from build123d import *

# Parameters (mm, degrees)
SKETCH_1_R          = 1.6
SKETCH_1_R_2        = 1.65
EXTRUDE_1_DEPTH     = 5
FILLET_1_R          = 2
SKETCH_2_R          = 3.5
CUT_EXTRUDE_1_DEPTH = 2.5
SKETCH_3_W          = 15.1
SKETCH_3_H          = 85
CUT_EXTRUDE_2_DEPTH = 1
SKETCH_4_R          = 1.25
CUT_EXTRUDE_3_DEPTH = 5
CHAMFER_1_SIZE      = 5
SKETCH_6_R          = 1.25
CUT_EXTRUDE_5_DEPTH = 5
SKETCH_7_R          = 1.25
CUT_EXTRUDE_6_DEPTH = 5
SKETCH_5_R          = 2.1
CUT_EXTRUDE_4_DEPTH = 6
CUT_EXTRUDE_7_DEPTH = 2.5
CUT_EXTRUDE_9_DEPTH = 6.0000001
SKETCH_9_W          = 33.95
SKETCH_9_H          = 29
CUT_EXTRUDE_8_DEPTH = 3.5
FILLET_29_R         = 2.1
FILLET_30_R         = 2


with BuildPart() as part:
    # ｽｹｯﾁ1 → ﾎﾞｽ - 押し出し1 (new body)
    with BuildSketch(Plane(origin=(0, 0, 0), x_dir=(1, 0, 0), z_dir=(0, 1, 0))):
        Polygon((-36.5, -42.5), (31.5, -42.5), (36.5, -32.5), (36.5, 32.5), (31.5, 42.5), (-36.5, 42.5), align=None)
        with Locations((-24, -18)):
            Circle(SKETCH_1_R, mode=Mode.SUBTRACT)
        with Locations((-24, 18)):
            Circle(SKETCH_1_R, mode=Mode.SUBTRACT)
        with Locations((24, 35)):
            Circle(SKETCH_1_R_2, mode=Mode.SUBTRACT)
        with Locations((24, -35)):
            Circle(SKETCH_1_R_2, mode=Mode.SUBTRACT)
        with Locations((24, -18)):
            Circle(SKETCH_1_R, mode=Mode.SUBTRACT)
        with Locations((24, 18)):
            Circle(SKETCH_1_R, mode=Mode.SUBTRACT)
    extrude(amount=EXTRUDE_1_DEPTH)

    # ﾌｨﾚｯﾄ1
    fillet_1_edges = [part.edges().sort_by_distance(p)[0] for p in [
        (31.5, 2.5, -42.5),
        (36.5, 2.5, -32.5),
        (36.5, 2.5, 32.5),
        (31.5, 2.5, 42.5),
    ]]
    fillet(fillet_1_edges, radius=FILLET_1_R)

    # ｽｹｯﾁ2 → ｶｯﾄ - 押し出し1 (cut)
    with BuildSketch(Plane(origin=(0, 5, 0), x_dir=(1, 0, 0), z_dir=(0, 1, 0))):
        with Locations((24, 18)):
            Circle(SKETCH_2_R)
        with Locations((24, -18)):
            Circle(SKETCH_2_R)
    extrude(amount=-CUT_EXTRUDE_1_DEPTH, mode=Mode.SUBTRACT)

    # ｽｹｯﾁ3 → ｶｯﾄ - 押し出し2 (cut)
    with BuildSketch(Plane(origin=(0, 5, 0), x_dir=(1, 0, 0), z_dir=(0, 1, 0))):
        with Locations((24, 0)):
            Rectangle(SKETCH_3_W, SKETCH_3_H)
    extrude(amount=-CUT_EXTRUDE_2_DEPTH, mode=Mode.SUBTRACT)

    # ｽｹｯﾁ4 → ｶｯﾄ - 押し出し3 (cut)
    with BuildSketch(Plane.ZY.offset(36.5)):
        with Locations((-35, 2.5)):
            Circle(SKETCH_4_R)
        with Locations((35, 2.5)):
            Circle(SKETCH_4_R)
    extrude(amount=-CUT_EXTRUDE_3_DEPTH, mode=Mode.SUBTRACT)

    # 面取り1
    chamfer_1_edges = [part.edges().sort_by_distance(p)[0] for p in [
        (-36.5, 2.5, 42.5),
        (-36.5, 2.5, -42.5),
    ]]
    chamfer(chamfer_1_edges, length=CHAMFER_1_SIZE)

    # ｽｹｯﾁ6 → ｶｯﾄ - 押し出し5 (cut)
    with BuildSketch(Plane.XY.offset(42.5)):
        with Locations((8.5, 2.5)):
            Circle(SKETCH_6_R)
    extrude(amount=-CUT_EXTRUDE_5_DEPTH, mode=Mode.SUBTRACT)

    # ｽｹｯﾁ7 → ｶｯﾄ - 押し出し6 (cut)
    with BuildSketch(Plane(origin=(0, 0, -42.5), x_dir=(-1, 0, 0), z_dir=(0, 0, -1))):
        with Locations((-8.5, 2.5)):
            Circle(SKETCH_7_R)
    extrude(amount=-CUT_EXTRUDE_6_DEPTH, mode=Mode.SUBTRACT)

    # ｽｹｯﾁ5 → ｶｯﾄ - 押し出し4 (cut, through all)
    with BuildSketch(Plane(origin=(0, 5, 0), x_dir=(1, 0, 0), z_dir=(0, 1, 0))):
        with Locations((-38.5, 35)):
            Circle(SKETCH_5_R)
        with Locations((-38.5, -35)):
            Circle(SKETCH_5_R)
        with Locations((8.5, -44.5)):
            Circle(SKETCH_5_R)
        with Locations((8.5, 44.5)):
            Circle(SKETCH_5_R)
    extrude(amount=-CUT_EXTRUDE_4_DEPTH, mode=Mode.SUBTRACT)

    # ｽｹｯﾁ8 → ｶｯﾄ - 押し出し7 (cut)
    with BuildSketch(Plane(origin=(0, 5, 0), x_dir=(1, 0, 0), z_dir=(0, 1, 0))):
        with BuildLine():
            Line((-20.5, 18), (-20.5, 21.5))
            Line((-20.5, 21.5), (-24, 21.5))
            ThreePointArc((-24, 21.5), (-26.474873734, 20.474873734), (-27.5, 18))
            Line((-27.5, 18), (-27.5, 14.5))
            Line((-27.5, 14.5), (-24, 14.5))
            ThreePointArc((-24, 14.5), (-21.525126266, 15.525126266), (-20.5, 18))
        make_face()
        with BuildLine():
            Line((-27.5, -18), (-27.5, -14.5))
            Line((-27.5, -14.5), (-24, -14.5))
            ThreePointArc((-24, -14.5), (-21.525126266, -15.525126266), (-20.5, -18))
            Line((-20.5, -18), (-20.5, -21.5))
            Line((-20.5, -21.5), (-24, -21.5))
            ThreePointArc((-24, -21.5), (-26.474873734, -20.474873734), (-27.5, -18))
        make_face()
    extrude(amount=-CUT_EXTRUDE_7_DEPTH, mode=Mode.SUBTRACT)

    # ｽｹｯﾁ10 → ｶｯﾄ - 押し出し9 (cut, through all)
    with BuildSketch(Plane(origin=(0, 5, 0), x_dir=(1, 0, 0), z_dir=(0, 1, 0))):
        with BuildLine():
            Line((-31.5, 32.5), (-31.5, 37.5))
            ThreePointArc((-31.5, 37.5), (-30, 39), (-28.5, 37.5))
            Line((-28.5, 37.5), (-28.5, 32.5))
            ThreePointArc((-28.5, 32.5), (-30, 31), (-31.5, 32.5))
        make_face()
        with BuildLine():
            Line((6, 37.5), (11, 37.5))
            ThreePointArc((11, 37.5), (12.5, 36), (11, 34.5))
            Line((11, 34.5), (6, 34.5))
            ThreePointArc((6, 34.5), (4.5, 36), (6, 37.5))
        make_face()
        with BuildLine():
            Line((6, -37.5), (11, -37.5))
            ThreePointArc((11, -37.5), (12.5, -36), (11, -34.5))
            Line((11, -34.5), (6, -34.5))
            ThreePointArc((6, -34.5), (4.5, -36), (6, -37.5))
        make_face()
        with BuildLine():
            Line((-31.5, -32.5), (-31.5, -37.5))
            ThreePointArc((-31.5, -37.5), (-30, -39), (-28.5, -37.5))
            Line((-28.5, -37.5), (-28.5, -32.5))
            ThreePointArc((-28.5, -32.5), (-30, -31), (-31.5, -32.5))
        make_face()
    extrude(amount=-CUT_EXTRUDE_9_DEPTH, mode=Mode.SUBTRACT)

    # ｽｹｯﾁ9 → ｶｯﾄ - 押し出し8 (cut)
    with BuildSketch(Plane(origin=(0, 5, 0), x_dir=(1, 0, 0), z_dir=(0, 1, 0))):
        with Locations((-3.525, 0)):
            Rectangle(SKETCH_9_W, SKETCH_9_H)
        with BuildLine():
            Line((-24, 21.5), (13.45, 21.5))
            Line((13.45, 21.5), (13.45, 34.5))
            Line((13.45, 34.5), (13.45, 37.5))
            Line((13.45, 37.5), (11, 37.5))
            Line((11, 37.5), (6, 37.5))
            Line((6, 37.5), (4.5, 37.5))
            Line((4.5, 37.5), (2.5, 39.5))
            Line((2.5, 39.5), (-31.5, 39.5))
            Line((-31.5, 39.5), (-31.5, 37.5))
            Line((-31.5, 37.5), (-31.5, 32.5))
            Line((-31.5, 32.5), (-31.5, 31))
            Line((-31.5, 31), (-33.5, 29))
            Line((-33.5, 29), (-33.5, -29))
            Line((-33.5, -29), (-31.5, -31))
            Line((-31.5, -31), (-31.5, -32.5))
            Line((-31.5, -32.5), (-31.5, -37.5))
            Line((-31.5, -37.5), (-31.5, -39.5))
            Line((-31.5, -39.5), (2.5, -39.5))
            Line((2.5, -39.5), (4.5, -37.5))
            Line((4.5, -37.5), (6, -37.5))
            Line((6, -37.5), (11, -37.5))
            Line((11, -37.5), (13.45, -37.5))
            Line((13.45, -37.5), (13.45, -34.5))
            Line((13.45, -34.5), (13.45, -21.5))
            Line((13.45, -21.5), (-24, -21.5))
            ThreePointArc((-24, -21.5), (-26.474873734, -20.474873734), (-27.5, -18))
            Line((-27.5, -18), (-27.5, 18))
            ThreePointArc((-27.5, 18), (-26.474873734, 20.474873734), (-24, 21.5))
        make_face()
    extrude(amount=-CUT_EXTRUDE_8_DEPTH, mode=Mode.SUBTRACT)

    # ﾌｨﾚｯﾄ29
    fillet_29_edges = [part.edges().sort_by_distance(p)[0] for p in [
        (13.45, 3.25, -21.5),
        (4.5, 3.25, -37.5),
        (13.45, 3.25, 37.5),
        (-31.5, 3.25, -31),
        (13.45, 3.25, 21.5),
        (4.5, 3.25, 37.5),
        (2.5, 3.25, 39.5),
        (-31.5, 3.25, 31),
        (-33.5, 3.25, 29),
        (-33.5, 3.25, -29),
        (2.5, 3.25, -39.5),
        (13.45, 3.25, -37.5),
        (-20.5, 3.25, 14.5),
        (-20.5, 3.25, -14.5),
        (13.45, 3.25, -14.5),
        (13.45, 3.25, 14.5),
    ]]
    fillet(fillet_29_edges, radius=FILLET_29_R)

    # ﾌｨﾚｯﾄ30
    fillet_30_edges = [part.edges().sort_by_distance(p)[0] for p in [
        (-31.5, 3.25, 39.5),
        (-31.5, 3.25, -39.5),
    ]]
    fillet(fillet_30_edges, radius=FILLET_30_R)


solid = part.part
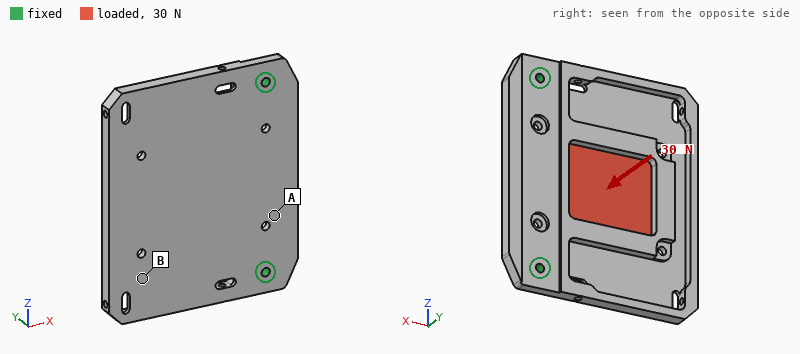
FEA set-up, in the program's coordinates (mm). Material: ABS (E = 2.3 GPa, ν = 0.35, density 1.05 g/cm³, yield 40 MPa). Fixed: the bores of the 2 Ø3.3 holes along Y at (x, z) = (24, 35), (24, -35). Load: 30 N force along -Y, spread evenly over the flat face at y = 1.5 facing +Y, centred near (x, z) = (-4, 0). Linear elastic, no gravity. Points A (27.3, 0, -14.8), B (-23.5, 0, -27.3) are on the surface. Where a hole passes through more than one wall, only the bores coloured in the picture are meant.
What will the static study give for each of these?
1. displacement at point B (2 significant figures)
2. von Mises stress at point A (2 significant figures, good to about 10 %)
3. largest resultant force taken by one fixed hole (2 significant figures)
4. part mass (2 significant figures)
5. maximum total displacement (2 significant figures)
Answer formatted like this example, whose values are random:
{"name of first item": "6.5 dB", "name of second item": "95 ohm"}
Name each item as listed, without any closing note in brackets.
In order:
{"displacement at point B": "0.92 mm", "von Mises stress at point A": "2.1 MPa", "largest resultant force taken by one fixed hole": "15 N", "part mass": "20 g", "maximum total displacement": "1.3 mm"}
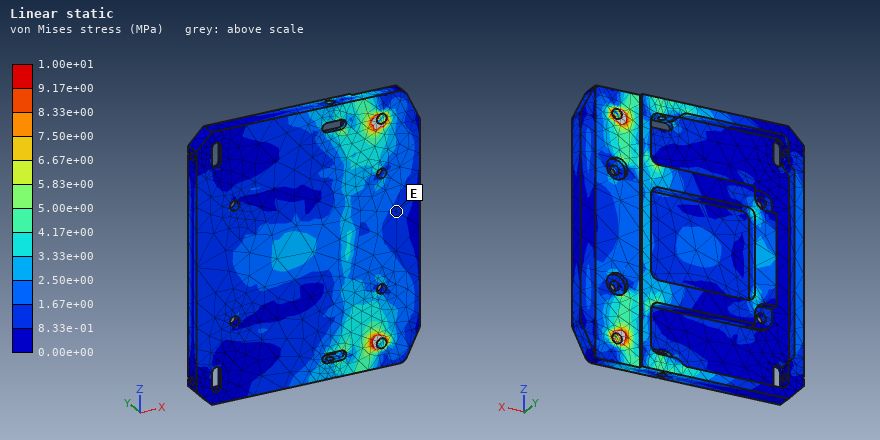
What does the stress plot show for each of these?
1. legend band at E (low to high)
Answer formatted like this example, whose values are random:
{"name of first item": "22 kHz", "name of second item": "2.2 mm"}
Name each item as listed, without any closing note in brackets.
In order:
{"legend band at E": "8.33e-01 to 1.67e+00 MPa"}
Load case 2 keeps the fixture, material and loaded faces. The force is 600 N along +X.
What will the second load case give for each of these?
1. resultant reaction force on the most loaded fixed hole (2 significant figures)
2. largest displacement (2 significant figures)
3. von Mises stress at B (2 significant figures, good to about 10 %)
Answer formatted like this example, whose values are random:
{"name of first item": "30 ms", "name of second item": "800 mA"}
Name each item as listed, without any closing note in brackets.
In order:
{"resultant reaction force on the most loaded fixed hole": "310 N", "largest displacement": "0.45 mm", "von Mises stress at B": "2.0 MPa"}
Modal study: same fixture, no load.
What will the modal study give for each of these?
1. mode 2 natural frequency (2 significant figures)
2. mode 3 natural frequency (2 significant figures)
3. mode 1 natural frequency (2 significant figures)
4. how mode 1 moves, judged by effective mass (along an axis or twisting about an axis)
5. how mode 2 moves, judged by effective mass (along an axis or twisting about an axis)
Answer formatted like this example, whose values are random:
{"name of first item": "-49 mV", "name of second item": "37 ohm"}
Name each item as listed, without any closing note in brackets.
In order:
{"mode 2 natural frequency": "450 Hz", "mode 3 natural frequency": "980 Hz", "mode 1 natural frequency": "240 Hz", "how mode 1 moves, judged by effective mass": "along Y", "how mode 2 moves, judged by effective mass": "twisting about X"}
